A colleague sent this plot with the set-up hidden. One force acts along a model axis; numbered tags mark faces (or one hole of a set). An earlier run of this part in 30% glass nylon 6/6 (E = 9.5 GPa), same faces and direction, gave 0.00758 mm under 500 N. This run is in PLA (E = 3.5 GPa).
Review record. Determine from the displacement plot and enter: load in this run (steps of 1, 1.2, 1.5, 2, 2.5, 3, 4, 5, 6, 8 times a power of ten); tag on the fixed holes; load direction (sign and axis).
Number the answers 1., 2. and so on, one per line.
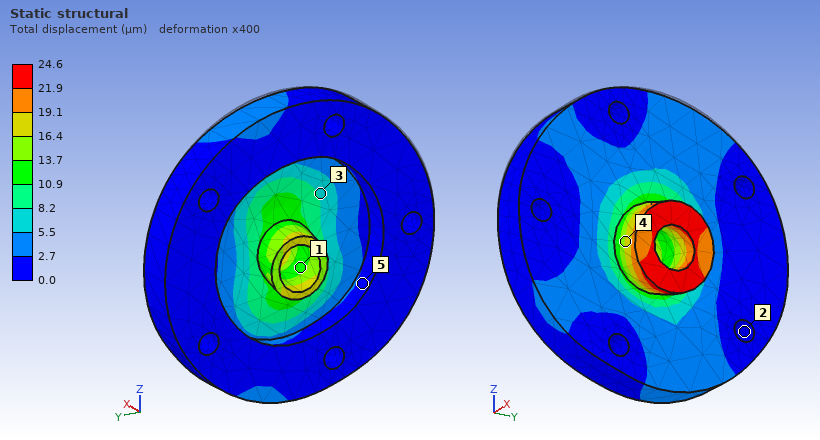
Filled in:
1. 600 N
2. 2
3. -Z
